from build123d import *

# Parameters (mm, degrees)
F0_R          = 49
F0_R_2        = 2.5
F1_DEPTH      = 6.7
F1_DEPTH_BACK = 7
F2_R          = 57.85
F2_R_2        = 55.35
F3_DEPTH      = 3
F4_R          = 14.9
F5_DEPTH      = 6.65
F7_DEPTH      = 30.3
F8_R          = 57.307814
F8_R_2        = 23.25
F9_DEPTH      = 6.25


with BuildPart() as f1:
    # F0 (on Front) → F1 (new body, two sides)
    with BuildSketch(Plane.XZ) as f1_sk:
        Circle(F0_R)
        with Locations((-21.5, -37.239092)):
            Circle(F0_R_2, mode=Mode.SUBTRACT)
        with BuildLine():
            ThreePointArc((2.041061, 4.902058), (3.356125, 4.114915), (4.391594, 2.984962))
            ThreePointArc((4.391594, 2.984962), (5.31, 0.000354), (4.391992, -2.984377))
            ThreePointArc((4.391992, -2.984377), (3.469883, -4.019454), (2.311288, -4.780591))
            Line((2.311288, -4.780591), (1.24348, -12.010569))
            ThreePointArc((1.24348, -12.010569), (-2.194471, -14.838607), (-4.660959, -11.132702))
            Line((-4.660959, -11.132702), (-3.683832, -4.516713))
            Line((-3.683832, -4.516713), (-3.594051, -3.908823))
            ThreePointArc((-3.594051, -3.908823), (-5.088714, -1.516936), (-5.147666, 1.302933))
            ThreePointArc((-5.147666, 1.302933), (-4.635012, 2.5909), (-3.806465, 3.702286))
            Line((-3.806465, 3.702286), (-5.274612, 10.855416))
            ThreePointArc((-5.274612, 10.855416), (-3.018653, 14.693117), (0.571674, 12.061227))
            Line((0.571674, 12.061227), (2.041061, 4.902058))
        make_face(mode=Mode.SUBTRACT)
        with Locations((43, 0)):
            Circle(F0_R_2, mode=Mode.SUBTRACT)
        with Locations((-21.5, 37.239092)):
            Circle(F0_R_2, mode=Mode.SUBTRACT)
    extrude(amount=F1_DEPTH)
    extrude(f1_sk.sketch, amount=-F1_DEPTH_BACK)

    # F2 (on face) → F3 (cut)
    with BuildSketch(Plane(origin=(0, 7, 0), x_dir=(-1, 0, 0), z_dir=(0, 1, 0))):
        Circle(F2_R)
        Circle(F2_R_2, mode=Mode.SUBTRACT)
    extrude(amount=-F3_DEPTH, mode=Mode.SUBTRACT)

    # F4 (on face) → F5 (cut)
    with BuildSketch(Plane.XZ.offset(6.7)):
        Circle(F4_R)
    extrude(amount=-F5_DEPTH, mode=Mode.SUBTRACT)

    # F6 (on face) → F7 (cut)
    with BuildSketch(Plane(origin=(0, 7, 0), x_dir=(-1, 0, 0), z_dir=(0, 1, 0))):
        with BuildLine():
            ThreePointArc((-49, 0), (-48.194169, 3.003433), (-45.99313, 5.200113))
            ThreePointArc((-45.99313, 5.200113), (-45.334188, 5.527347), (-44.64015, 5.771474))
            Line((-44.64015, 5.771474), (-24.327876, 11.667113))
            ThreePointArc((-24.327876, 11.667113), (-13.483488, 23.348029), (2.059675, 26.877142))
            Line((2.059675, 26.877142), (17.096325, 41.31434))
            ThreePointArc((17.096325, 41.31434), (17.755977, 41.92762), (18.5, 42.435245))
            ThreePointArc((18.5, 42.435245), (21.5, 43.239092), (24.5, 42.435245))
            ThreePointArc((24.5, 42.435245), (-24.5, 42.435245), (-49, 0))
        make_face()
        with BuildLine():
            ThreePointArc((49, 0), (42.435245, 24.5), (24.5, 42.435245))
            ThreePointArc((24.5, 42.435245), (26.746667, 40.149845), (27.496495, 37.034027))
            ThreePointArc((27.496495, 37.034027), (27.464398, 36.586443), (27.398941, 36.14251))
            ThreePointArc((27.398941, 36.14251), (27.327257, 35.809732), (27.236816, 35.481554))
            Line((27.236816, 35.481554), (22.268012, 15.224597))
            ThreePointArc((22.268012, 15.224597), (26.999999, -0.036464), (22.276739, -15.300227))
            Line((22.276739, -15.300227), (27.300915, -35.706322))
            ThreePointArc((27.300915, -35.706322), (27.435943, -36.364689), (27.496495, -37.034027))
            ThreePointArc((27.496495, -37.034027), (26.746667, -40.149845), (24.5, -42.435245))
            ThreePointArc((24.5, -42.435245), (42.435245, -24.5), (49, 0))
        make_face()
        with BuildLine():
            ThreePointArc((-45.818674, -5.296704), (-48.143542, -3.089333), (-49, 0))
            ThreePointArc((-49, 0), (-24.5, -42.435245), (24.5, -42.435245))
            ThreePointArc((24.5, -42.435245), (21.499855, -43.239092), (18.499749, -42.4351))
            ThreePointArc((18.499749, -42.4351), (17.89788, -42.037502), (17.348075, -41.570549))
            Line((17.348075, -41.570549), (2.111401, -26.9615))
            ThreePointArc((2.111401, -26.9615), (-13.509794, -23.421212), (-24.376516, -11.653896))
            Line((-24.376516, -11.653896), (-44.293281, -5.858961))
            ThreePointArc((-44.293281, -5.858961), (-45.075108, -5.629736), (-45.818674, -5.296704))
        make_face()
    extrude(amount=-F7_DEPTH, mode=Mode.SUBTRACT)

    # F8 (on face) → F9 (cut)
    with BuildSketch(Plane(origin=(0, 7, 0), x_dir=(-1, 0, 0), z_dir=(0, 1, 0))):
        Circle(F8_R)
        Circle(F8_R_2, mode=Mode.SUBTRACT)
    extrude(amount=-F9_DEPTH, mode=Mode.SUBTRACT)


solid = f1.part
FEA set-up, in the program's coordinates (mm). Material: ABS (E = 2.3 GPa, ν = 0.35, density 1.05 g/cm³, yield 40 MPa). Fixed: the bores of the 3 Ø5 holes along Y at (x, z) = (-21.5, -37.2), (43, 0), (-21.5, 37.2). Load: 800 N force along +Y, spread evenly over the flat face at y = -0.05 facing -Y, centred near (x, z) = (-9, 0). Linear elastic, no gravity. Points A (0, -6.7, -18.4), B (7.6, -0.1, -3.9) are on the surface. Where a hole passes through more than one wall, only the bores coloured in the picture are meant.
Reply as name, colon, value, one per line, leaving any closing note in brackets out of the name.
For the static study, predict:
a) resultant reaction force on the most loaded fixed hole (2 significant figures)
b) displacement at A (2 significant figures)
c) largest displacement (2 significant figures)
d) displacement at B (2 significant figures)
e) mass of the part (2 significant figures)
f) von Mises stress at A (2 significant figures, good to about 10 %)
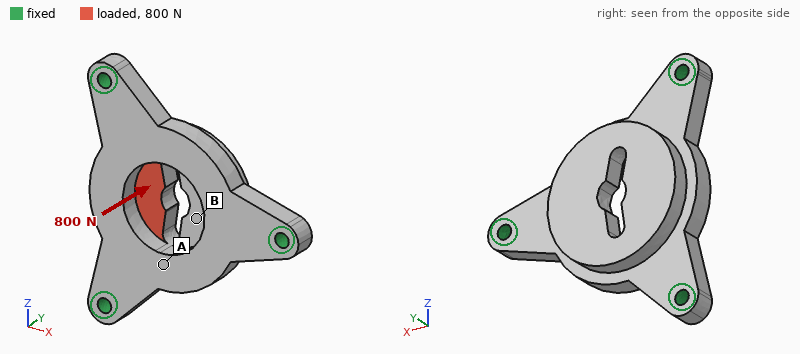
resultant reaction force on the most loaded fixed hole: 440 N
displacement at A: 0.33 mm
largest displacement: 0.58 mm
displacement at B: 0.30 mm
mass of the part: 30 g
von Mises stress at A: 8.6 MPa
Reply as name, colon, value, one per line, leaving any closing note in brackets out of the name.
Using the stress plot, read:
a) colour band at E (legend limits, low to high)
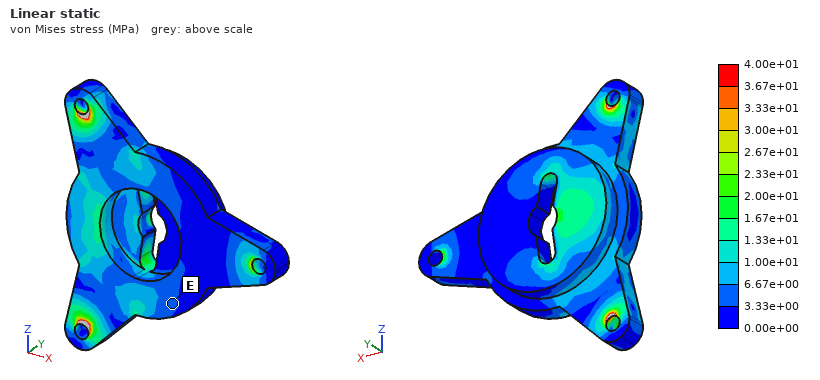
colour band at E: 3.33e+00 to 6.67e+00 MPa
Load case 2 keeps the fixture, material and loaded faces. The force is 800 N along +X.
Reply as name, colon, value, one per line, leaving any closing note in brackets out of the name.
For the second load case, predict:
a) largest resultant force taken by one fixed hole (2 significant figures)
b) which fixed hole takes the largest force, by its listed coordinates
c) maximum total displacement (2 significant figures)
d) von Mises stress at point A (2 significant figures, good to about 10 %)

largest resultant force taken by one fixed hole: 370 N
which fixed hole takes the largest force, by its listed coordinates: (43, 0)
maximum total displacement: 0.19 mm
von Mises stress at point A: 3.0 MPa
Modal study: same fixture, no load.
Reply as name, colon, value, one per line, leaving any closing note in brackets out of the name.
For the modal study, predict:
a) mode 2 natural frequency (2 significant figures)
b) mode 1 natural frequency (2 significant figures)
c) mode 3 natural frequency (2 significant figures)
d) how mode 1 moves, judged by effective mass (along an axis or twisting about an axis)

mode 2 natural frequency: 2500 Hz
mode 1 natural frequency: 1700 Hz
mode 3 natural frequency: 2500 Hz
how mode 1 moves, judged by effective mass: along Y
